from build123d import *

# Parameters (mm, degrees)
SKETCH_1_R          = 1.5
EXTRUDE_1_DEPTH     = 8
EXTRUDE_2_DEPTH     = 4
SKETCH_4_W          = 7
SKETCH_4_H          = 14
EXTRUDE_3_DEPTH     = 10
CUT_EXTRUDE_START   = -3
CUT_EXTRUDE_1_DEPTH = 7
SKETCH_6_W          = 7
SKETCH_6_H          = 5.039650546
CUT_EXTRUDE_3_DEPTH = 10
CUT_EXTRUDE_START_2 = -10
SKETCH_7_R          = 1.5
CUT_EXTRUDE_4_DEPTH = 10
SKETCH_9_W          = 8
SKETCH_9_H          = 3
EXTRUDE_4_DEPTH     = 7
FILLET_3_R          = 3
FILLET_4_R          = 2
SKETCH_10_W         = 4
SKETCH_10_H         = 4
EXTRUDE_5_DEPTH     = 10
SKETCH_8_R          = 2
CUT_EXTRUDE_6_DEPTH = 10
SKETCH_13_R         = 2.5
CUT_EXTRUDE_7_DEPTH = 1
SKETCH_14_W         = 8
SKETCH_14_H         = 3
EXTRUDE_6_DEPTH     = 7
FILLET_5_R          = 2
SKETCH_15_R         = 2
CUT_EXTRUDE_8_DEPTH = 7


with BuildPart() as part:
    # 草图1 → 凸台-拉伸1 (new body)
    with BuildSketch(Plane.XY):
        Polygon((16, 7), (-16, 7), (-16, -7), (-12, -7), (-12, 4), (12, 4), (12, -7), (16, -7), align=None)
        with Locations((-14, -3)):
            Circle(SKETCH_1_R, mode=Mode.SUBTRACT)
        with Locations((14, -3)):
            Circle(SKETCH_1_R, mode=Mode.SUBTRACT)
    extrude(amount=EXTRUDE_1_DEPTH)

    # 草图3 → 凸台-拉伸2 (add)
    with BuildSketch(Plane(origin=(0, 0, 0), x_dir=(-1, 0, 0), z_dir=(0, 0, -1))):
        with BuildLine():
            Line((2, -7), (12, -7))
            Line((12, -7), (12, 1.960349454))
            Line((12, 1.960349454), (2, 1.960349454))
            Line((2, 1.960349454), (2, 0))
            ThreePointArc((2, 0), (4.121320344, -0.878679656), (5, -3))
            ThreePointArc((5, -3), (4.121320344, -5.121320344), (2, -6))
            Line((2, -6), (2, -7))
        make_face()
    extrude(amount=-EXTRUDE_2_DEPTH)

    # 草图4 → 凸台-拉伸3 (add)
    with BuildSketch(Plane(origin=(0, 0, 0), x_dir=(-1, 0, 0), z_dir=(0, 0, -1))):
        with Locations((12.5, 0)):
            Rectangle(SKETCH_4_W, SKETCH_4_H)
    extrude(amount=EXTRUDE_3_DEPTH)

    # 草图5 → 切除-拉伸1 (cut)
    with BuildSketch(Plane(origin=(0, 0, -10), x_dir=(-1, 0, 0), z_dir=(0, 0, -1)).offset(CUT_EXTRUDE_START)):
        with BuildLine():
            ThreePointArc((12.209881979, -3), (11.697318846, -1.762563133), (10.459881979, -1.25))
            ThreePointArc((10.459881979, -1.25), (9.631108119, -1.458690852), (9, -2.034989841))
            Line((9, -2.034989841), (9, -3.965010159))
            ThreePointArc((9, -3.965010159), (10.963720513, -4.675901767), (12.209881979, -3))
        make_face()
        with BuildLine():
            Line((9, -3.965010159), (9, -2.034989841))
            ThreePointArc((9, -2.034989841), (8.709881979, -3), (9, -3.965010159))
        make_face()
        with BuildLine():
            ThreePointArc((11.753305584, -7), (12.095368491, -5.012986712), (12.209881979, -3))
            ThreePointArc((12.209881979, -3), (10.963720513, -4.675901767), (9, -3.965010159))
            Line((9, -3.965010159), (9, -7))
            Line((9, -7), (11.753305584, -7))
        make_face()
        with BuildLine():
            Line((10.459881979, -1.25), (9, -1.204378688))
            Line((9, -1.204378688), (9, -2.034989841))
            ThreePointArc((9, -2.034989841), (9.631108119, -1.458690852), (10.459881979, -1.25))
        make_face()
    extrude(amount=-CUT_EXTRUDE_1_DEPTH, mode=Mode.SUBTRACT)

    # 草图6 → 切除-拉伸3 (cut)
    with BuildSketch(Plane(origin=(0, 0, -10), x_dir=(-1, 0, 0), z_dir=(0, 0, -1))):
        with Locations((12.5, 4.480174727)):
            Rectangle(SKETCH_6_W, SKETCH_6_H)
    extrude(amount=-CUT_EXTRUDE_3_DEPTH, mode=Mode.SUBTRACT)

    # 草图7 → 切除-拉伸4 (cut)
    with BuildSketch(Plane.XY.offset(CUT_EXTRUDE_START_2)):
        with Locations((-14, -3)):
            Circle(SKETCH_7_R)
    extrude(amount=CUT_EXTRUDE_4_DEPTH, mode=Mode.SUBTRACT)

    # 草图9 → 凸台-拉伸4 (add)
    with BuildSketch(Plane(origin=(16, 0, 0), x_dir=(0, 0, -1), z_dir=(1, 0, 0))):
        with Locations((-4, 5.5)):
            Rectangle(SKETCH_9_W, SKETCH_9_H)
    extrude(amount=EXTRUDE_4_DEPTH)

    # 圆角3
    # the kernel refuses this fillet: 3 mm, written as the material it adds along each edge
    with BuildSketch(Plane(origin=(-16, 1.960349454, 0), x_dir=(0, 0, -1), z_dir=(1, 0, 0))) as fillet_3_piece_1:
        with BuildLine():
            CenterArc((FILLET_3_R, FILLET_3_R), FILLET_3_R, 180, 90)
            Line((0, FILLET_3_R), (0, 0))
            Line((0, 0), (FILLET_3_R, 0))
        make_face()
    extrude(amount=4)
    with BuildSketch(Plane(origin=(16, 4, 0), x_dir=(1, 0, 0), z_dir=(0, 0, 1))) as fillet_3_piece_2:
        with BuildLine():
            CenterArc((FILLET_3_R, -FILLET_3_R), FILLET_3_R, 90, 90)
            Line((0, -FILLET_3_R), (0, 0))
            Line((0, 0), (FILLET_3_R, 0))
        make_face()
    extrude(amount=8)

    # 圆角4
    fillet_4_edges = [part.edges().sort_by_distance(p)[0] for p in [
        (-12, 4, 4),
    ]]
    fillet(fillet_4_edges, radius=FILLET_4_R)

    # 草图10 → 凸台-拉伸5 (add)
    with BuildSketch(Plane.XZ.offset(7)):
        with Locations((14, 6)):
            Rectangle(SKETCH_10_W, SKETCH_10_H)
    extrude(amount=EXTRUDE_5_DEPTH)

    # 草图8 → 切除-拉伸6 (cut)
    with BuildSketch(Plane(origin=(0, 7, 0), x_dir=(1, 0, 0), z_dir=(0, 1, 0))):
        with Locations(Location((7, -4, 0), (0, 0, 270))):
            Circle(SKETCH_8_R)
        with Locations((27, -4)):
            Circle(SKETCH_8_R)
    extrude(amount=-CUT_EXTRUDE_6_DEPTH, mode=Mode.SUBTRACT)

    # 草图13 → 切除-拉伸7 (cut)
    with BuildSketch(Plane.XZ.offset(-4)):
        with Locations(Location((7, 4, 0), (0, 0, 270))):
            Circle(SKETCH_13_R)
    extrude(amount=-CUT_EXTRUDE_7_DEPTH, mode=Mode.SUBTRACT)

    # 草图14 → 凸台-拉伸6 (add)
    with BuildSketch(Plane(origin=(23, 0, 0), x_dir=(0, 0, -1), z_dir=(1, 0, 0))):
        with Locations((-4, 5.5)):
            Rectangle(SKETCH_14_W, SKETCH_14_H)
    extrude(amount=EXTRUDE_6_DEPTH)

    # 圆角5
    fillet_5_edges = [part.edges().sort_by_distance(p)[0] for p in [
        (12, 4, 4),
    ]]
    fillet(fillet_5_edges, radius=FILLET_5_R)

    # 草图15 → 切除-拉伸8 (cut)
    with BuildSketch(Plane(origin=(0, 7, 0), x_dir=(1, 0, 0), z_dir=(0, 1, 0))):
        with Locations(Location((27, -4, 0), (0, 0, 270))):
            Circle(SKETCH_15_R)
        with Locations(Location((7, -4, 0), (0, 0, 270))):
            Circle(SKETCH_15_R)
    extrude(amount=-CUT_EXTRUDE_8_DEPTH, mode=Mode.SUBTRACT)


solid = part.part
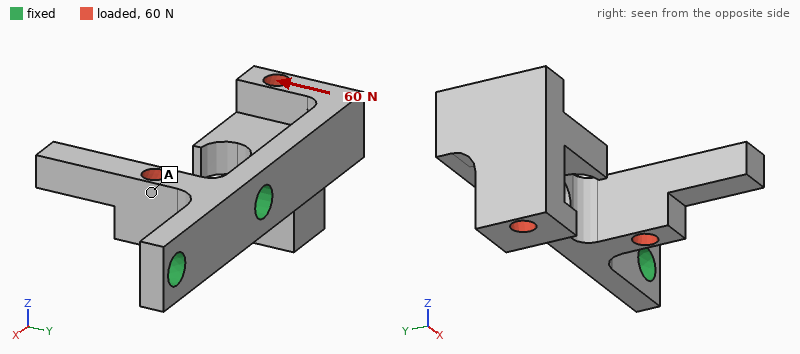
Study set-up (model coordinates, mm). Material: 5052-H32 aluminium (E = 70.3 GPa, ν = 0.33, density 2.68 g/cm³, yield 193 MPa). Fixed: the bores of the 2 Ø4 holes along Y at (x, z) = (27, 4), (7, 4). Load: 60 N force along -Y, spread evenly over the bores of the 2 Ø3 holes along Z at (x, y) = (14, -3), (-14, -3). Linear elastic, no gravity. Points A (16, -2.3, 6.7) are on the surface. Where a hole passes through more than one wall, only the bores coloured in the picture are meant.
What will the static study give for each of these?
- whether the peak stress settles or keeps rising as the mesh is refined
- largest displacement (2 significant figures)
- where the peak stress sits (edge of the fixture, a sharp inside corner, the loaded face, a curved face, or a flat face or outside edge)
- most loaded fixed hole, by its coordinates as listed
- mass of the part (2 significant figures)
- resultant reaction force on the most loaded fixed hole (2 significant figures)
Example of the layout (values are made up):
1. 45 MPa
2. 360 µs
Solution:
1. keeps rising
2. 0.18 mm
3. edge of the fixture
4. (7, 4)
5. 6.8 g
6. 58 N
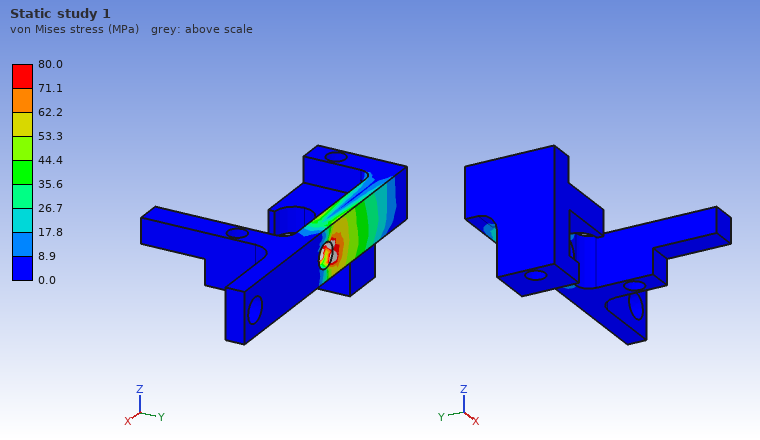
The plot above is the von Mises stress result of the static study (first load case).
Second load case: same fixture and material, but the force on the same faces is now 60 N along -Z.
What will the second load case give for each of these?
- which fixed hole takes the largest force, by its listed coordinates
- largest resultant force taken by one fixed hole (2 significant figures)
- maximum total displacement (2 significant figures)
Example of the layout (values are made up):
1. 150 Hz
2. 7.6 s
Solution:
1. (7, 4)
2. 65 N
3. 95 µm
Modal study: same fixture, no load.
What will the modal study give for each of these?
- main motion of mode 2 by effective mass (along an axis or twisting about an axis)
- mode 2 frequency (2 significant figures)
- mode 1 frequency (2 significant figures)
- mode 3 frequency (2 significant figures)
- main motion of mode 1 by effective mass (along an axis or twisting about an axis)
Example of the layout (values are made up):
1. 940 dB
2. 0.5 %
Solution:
1. along Z
2. 2600 Hz
3. 1700 Hz
4. 5500 Hz
5. along Y
